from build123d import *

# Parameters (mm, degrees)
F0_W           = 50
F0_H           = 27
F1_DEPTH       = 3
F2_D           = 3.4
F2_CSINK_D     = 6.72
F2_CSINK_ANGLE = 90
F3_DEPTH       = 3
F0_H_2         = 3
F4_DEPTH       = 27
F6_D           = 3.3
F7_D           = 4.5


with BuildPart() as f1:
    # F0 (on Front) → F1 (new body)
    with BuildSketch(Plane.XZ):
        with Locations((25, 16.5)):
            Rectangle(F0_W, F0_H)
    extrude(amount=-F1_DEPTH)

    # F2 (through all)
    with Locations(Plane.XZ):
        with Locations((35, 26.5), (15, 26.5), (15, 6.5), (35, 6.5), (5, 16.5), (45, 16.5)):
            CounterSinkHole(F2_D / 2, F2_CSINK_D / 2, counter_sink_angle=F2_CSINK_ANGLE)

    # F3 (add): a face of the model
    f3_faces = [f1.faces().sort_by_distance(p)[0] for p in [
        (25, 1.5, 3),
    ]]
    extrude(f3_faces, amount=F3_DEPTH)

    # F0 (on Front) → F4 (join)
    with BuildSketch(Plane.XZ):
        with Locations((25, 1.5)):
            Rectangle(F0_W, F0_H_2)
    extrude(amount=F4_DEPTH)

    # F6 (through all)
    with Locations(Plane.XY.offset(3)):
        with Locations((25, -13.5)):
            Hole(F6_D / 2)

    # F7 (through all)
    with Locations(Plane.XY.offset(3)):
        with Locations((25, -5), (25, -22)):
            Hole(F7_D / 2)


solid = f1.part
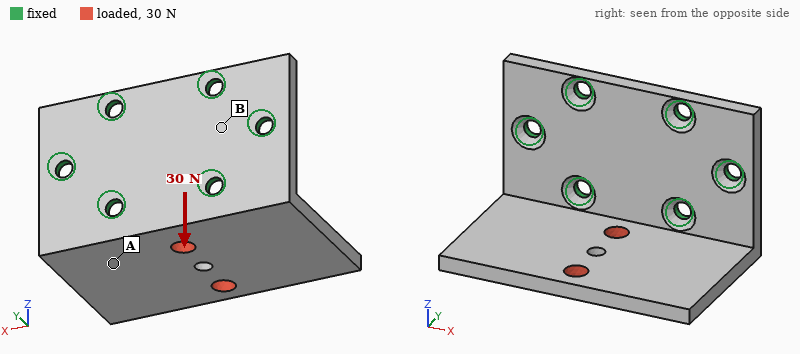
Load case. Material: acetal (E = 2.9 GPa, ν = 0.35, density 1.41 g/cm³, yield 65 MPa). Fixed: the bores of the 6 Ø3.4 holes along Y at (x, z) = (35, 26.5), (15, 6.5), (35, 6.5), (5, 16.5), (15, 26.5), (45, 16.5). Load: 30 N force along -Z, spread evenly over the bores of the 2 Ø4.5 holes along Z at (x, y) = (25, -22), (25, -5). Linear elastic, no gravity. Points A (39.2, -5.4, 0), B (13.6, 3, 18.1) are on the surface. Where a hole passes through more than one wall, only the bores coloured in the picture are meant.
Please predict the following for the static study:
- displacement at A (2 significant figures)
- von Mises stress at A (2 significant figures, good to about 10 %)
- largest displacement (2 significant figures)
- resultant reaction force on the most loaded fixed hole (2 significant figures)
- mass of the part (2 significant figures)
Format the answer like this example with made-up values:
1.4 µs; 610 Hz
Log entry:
0.11 mm; 3.5 MPa; 0.59 mm; 15 N; 11 g
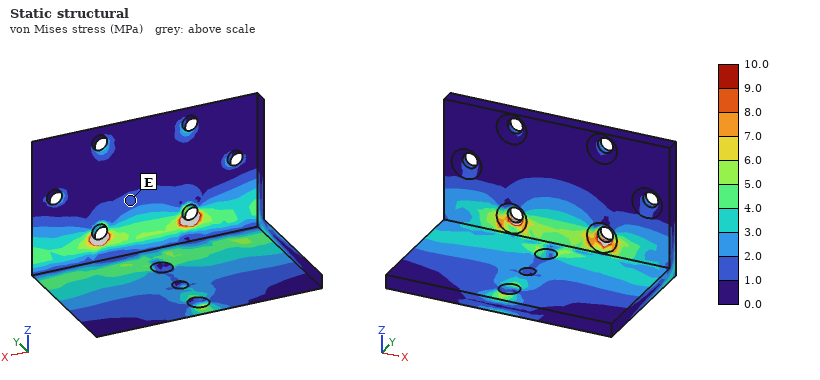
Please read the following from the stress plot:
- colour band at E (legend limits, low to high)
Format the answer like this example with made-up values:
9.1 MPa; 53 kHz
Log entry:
1.0 to 2.0 MPa
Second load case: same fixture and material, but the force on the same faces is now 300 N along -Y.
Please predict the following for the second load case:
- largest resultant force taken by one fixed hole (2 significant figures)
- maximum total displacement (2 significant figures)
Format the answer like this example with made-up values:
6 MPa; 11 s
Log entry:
180 N; 0.70 mm
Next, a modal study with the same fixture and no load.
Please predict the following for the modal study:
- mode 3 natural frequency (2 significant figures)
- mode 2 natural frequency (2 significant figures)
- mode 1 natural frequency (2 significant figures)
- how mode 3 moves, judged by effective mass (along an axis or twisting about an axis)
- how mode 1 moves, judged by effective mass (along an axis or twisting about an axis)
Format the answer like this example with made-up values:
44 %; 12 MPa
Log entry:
2000 Hz; 1100 Hz; 630 Hz; along X; along Z
